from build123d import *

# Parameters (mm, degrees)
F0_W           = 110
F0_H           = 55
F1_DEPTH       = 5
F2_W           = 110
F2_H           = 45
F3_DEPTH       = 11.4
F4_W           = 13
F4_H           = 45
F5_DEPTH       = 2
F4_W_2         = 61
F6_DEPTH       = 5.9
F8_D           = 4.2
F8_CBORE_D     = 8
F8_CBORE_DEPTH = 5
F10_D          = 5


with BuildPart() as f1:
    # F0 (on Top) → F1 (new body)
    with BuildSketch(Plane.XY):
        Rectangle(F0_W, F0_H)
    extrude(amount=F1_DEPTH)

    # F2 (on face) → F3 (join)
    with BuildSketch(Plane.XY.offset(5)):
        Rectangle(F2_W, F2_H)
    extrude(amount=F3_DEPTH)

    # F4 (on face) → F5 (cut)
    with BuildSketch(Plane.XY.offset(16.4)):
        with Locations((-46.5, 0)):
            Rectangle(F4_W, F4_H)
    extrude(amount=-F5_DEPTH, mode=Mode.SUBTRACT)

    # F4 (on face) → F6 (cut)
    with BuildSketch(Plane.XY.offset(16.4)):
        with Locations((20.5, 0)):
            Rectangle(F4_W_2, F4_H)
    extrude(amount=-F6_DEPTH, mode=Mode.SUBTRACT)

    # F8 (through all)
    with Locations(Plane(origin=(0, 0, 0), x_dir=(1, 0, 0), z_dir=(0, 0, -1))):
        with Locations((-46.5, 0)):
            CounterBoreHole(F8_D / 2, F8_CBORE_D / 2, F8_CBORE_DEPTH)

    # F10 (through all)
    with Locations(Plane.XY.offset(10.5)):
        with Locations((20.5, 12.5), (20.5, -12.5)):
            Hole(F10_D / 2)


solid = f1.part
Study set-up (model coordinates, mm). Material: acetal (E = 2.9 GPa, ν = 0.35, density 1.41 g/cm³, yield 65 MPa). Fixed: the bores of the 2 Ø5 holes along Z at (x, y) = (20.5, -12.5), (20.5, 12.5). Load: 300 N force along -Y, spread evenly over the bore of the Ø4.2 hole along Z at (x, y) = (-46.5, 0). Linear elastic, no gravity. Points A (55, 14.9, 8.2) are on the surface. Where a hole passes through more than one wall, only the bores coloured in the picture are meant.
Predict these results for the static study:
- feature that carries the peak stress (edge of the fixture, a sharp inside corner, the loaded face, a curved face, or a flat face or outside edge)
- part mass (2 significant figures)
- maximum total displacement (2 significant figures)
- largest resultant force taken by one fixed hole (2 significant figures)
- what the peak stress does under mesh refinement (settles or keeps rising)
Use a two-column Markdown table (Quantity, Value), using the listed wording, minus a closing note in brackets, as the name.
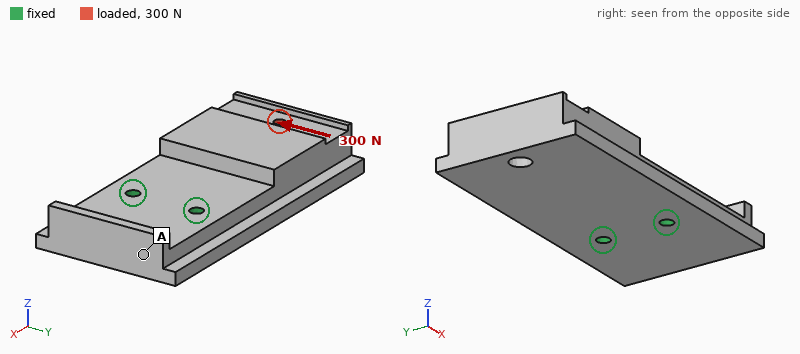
| Quantity | Value |
|---|---|
| feature that carries the peak stress | edge of the fixture |
| part mass | 97 g |
| maximum total displacement | 0.21 mm |
| largest resultant force taken by one fixed hole | 740 N |
| what the peak stress does under mesh refinement | keeps rising |
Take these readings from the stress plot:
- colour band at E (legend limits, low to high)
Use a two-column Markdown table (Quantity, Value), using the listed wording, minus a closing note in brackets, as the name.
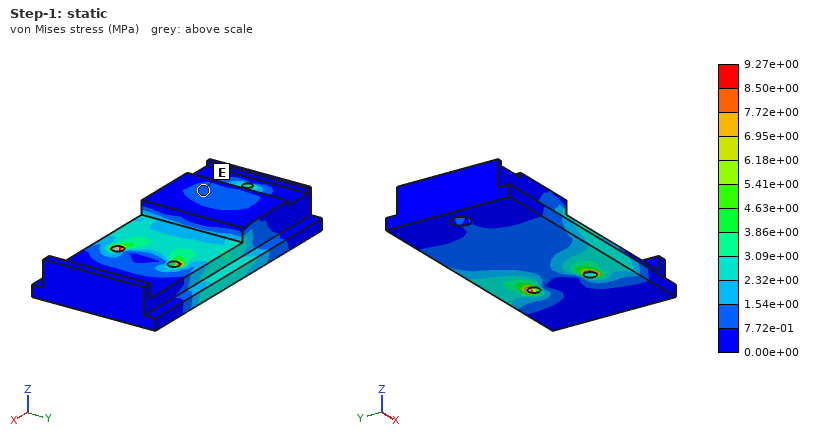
| Quantity | Value |
|---|---|
| colour band at E | 7.72e-01 to 1.54e+00 MPa |
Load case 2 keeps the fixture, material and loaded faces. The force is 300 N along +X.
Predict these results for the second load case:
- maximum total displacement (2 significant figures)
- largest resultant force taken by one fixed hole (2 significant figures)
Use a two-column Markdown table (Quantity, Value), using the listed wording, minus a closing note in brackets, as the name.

| Quantity | Value |
|---|---|
| maximum total displacement | 0.22 mm |
| largest resultant force taken by one fixed hole | 150 N |
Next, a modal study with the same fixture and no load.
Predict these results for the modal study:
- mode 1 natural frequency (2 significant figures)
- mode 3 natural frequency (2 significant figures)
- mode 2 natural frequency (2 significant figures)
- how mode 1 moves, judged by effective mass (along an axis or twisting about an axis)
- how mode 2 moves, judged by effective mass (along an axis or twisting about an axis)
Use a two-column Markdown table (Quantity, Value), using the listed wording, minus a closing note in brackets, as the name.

| Quantity | Value |
|---|---|
| mode 1 natural frequency | 360 Hz |
| mode 3 natural frequency | 1200 Hz |
| mode 2 natural frequency | 1200 Hz |
| how mode 1 moves, judged by effective mass | along Z |
| how mode 2 moves, judged by effective mass | along Y |
